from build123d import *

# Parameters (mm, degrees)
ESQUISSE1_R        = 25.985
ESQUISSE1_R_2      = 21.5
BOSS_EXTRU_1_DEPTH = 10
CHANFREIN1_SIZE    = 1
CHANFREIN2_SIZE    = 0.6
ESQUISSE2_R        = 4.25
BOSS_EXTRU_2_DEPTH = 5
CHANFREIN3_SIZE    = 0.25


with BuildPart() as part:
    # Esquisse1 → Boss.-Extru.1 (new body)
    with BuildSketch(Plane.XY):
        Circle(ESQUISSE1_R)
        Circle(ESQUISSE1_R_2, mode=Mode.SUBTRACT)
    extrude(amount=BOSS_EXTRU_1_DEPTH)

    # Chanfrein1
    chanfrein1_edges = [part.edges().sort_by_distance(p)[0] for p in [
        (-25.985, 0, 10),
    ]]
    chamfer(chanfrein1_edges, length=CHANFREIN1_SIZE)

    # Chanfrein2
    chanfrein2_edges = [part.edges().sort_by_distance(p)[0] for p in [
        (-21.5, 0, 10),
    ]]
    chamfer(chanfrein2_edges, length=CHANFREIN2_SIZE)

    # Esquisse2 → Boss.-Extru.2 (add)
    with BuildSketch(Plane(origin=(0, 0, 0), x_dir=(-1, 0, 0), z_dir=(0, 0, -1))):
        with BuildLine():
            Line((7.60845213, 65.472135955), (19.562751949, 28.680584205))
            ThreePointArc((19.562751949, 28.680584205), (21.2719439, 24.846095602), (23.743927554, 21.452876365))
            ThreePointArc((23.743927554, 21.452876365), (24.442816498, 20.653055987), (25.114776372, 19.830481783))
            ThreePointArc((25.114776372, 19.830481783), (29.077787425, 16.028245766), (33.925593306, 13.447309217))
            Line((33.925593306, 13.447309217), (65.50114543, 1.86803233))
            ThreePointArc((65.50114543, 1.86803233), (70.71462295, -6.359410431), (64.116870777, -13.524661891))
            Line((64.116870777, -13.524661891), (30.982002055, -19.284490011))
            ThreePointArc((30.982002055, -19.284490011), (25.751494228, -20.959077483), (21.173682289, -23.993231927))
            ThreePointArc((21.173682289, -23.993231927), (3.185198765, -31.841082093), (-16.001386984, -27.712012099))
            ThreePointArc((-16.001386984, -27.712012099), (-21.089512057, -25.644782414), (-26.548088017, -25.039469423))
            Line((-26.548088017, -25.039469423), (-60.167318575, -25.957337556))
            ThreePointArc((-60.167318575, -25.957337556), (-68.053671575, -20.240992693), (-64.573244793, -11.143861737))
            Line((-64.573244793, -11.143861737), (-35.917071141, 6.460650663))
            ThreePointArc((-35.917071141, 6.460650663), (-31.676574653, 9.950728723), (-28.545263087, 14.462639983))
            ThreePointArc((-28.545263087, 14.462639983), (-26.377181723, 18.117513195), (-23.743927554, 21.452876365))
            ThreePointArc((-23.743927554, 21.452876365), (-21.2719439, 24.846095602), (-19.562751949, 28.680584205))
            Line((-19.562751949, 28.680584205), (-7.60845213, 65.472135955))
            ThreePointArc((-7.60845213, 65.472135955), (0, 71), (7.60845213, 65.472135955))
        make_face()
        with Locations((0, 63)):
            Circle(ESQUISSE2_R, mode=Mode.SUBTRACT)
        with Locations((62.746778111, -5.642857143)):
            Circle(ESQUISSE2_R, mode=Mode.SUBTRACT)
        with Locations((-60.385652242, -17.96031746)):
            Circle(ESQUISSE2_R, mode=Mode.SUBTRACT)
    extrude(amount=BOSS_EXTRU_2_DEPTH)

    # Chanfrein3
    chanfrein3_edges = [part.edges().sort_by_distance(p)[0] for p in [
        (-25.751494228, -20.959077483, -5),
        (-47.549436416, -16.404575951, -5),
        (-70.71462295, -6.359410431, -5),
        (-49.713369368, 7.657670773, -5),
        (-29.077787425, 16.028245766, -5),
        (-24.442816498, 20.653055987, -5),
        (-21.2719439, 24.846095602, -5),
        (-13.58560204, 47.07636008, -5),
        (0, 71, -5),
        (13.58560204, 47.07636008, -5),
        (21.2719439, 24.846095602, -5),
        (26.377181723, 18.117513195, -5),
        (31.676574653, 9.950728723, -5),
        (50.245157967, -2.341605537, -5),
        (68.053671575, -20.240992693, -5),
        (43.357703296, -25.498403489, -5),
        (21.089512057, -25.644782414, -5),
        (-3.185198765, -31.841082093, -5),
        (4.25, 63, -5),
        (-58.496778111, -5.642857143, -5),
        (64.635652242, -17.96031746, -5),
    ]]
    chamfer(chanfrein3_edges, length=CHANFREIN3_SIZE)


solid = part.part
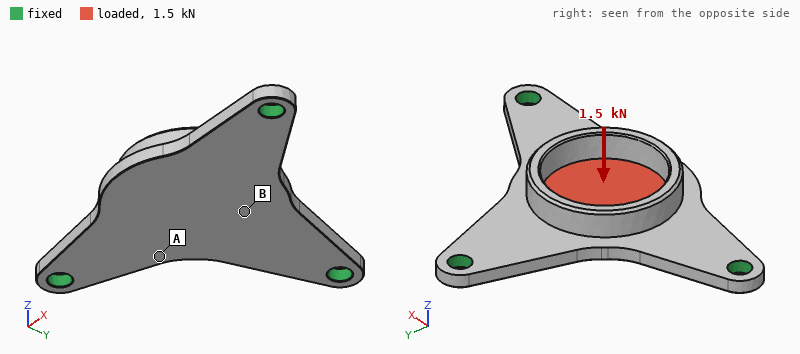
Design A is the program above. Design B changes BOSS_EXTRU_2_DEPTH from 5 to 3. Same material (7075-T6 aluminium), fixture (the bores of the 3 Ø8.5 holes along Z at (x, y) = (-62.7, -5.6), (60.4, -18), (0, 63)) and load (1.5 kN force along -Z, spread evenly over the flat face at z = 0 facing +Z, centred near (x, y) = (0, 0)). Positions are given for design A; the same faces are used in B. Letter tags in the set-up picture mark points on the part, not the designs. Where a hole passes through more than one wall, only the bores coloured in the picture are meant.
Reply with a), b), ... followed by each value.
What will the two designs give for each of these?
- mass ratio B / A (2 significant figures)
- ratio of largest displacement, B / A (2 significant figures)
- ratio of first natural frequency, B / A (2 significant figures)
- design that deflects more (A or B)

a) 0.67
b) 3.4
c) 0.63
d) B
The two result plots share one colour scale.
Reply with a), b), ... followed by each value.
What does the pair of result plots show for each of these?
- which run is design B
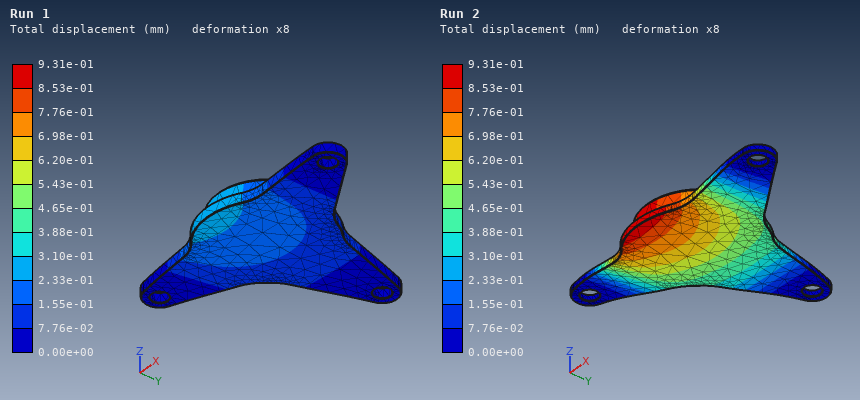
a) Run 2
